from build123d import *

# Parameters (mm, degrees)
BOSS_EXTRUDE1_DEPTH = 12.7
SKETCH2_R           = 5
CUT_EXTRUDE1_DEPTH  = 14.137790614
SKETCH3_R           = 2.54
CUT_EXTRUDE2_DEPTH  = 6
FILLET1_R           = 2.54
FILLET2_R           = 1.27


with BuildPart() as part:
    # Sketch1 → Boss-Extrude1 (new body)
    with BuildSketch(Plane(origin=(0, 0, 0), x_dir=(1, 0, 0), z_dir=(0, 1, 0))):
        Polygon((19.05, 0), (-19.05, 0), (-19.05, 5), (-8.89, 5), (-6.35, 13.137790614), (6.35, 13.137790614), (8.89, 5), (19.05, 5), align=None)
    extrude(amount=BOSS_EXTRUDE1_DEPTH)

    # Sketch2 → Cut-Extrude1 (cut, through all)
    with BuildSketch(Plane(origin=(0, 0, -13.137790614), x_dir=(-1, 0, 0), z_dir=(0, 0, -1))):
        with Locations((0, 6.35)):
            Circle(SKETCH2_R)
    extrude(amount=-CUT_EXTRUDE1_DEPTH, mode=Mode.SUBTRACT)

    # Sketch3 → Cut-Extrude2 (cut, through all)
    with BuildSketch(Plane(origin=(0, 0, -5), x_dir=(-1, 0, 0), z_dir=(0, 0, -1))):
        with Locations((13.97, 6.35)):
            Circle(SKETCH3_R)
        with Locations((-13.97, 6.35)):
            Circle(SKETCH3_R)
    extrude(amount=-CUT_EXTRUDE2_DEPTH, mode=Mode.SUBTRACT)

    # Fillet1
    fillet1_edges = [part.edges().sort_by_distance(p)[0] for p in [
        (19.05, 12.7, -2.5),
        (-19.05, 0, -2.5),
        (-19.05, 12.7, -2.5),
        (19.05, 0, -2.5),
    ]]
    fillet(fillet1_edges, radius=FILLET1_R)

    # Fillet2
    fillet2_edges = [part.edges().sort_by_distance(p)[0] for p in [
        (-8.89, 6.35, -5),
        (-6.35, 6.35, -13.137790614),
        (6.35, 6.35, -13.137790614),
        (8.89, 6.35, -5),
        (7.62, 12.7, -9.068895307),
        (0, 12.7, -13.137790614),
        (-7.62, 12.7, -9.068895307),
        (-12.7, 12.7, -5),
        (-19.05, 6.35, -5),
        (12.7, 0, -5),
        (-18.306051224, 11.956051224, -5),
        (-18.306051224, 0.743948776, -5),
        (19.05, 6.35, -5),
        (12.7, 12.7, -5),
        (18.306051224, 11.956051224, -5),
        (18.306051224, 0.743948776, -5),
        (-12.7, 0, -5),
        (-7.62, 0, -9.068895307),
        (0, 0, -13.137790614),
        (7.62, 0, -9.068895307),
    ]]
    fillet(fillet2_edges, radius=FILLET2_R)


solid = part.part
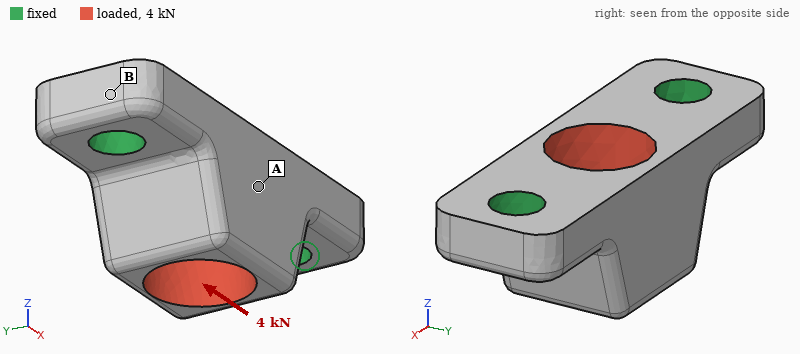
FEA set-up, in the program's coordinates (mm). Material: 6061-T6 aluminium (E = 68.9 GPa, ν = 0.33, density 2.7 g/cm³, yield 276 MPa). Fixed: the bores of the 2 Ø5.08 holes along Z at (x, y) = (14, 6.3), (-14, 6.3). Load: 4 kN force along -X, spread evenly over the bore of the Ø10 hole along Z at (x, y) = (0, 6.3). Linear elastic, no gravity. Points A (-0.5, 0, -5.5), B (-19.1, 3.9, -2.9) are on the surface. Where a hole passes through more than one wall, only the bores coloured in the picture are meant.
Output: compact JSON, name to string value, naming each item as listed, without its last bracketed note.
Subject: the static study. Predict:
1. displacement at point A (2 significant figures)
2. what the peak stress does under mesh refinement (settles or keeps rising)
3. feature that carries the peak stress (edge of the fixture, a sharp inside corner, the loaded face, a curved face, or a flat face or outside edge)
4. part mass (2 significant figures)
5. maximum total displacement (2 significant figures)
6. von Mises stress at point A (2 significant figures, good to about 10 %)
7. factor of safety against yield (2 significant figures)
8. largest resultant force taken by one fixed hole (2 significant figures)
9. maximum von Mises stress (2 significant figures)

{"displacement at point A": "6.3 µm", "what the peak stress does under mesh refinement": "settles", "feature that carries the peak stress": "a curved face", "part mass": "7.3 g", "maximum total displacement": "15 µm", "von Mises stress at point A": "44 MPa", "factor of safety against yield": "2.1", "largest resultant force taken by one fixed hole": "2.1 kN", "maximum von Mises stress": "130 MPa"}
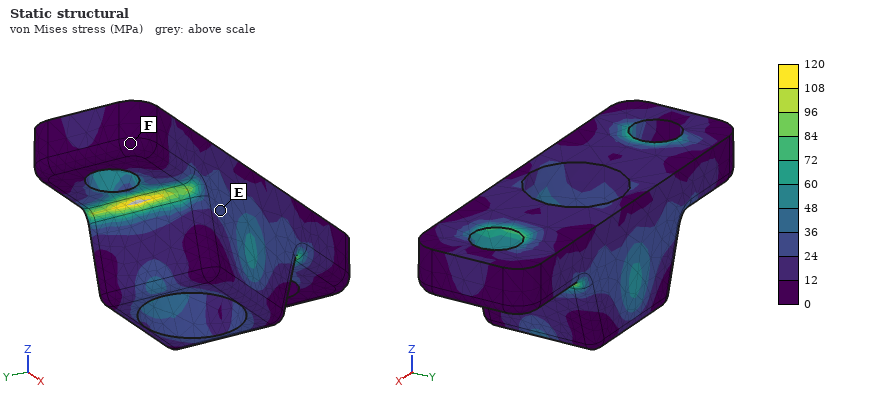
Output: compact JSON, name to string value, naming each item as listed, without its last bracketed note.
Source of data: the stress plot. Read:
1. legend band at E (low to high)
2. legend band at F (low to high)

{"legend band at E": "24 to 36 MPa", "legend band at F": "0 to 12 MPa"}
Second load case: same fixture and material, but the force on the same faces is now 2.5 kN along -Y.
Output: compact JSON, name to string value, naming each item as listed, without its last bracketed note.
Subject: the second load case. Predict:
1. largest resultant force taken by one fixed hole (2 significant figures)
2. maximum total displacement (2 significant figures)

{"largest resultant force taken by one fixed hole": "1.3 kN", "maximum total displacement": "42 µm"}
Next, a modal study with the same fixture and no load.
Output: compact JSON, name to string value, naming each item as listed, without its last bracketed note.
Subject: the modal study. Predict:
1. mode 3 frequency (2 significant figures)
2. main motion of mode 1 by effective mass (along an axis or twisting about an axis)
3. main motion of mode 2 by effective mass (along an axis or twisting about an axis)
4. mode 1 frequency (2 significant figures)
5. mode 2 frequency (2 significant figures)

{"mode 3 frequency": "41 kHz", "main motion of mode 1 by effective mass": "along Y", "main motion of mode 2 by effective mass": "along Z", "mode 1 frequency": "23 kHz", "mode 2 frequency": "35 kHz"}
